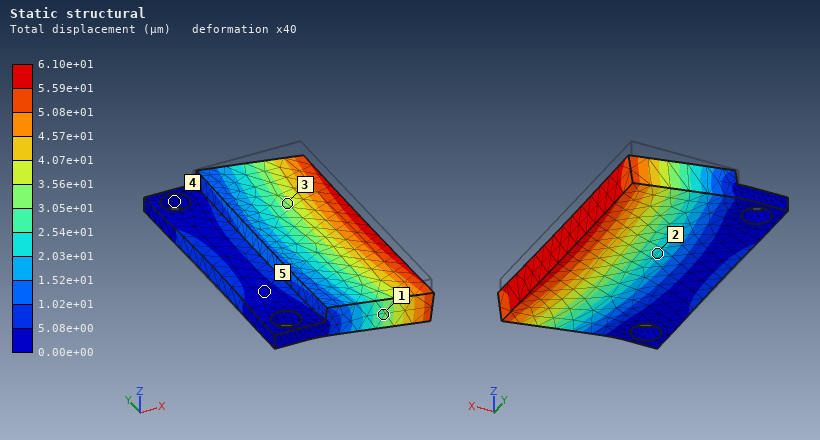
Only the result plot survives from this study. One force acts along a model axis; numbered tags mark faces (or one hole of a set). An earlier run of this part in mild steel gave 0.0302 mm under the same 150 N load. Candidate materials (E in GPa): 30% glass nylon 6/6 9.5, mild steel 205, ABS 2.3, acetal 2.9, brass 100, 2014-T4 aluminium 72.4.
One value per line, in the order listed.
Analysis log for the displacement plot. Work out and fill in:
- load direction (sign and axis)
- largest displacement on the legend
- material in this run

-Z
6.10e+01 µm
brass
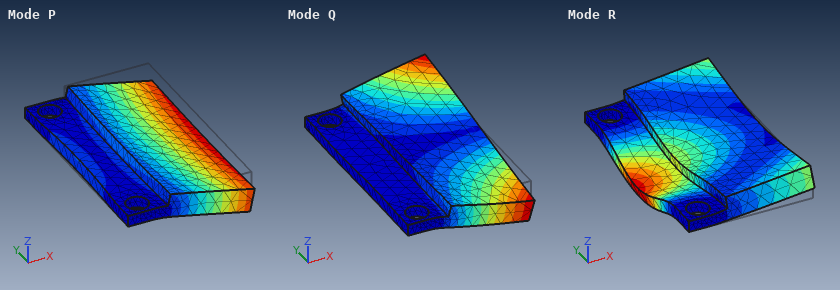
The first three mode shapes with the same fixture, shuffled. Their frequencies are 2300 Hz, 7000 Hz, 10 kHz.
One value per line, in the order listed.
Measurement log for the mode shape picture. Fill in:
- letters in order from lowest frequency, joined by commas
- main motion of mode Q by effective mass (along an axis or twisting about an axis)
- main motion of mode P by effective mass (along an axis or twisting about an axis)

P, Q, R
twisting about X
along Z
